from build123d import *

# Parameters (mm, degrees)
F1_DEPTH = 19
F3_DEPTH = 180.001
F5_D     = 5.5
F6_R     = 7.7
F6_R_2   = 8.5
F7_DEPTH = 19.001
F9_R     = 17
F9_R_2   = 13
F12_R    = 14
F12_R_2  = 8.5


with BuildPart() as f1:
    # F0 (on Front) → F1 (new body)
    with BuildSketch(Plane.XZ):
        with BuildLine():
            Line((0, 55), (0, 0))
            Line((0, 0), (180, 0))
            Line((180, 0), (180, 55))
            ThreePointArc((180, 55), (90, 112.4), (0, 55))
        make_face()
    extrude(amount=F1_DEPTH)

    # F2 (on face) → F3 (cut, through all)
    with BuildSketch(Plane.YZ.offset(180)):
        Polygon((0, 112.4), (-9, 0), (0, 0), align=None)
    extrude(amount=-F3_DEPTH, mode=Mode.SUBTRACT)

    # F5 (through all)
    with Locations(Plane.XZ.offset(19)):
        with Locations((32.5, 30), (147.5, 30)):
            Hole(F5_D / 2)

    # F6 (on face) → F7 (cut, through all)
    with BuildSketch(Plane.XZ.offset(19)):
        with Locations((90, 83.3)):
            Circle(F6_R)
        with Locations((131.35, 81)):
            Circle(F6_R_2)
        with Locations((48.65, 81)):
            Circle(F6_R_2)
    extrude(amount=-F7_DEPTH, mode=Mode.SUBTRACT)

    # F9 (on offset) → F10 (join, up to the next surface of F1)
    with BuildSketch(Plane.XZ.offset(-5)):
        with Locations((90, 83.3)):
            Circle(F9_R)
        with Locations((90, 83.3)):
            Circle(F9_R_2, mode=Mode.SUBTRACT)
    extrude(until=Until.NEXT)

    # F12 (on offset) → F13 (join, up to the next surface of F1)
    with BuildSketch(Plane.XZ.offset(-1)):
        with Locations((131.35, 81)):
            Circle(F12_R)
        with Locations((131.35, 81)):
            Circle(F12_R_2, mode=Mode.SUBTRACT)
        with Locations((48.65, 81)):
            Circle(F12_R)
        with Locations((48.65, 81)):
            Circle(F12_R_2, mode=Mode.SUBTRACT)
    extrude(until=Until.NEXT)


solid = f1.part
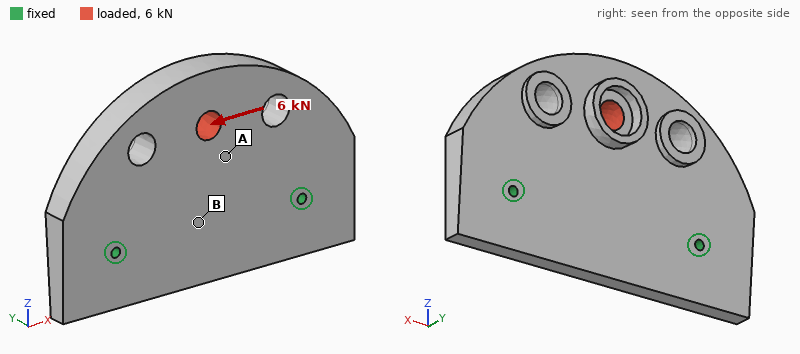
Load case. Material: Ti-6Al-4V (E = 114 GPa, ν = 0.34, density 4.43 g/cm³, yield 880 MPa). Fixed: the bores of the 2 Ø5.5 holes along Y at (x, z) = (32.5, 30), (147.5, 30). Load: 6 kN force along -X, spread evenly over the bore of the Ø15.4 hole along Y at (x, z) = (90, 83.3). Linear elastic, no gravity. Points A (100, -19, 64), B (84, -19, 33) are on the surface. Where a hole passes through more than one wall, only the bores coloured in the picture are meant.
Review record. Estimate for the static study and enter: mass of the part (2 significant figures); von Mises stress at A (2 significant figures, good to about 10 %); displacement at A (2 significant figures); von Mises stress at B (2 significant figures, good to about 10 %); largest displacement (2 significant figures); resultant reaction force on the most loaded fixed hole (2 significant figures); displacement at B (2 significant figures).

1.0 kg
7.0 MPa
4.6 µm
3.2 MPa
8.1 µm
4.1 kN
1.9 µm
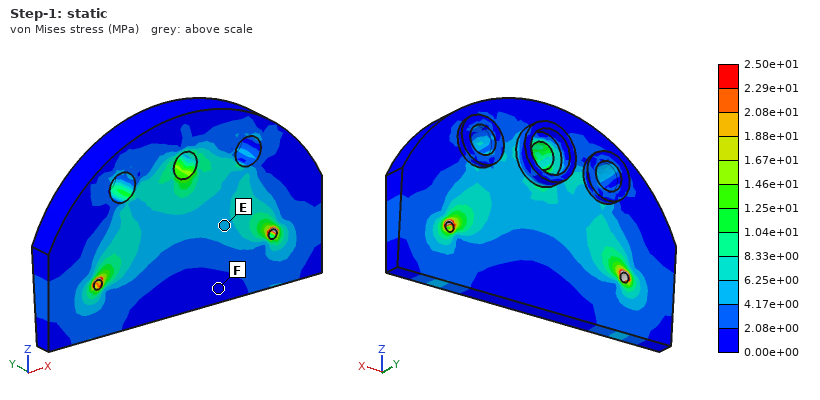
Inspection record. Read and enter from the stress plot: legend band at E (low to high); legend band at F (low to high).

4.17e+00 to 6.25e+00 MPa
0.00e+00 to 2.08e+00 MPa
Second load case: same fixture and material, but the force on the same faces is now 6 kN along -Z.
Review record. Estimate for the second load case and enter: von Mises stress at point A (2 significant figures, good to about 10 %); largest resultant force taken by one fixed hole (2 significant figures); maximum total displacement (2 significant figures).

4.9 MPa
3.2 kN
16 µm
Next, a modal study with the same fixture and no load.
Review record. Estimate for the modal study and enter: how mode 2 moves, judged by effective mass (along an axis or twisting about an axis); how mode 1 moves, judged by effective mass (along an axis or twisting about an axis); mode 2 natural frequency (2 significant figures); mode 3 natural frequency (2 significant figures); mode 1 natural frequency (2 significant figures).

twisting about Z
along Y
3200 Hz
3700 Hz
1200 Hz
